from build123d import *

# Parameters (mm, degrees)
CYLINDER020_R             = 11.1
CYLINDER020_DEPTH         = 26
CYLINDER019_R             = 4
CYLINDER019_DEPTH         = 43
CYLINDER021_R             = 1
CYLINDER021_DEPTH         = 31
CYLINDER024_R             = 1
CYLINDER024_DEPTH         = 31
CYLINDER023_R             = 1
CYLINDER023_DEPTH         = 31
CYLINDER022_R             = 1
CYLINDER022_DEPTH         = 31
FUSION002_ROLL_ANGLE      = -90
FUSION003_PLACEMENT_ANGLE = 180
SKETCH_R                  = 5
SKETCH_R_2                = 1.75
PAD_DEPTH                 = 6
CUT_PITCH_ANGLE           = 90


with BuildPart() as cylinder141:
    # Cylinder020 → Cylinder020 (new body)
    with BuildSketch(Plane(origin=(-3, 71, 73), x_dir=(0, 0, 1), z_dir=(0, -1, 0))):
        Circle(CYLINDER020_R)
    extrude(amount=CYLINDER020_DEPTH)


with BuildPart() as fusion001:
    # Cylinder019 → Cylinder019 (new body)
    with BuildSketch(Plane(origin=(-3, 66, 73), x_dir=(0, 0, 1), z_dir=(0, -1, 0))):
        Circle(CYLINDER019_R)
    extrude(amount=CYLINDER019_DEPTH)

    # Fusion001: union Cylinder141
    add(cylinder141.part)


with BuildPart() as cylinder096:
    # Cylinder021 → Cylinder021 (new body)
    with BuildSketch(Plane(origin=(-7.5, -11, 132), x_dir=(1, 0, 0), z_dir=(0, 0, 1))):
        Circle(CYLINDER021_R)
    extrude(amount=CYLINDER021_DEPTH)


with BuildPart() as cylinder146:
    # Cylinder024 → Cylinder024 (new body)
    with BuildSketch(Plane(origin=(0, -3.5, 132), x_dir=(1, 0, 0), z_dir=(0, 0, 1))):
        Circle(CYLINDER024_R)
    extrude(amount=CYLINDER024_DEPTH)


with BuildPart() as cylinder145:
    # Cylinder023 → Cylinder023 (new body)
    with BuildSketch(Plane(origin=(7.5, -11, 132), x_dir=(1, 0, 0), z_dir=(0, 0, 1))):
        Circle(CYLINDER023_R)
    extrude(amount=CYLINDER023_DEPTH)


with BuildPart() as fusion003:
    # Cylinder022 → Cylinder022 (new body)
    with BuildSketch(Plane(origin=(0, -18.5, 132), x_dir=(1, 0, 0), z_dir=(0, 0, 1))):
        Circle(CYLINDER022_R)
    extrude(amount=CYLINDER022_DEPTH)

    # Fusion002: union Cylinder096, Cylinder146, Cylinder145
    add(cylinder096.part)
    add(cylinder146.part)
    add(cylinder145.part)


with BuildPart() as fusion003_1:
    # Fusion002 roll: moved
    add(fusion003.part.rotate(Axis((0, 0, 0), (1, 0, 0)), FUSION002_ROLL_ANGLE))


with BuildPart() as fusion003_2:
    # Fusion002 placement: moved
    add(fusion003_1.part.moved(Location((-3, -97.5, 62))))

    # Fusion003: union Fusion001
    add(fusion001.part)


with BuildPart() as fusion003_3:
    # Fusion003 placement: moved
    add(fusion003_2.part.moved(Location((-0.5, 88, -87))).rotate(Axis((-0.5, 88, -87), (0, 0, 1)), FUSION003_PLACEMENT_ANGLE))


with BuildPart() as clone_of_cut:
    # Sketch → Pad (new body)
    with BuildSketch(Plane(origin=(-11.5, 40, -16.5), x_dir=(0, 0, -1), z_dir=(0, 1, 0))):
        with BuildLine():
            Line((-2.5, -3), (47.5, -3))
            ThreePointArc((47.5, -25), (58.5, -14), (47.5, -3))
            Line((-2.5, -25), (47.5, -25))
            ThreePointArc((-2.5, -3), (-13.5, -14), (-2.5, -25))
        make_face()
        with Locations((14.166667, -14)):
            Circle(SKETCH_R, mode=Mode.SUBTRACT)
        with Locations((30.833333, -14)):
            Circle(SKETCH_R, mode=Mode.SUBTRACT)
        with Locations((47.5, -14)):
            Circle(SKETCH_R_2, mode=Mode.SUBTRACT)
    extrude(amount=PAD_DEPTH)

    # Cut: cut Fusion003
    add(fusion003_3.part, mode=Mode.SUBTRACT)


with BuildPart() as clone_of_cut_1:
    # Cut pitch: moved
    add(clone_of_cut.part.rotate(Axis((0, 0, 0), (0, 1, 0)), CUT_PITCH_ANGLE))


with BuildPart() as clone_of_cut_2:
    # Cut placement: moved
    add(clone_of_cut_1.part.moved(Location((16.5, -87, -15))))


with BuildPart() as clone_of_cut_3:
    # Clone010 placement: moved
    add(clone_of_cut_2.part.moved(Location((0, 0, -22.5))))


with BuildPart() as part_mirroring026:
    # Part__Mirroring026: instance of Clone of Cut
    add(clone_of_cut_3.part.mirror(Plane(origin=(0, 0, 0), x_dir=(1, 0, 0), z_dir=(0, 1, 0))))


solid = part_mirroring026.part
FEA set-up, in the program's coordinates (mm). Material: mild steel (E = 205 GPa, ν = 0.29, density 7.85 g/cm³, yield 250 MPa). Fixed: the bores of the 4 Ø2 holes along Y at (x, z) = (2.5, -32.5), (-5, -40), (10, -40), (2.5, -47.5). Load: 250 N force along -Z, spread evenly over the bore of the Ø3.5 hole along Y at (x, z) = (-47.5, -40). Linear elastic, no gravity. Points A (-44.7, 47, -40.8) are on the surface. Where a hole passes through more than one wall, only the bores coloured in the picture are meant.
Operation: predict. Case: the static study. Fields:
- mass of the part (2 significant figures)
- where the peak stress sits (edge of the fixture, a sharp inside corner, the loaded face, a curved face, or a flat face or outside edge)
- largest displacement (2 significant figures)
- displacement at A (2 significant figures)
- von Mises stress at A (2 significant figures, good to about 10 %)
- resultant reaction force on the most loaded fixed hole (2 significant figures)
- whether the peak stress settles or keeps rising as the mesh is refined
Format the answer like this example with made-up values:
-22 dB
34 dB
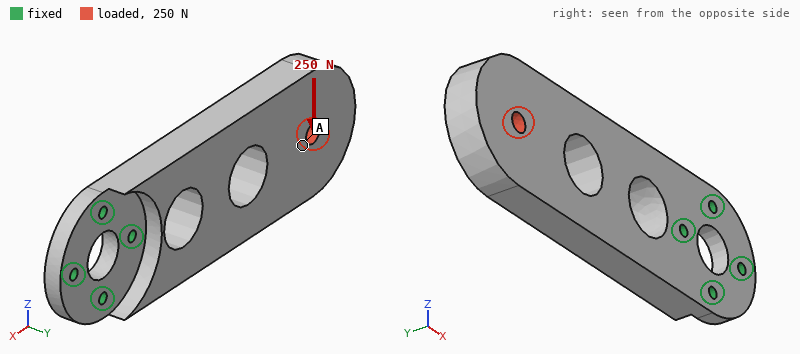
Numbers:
51 g
edge of the fixture
22 µm
15 µm
7.5 MPa
550 N
keeps rising
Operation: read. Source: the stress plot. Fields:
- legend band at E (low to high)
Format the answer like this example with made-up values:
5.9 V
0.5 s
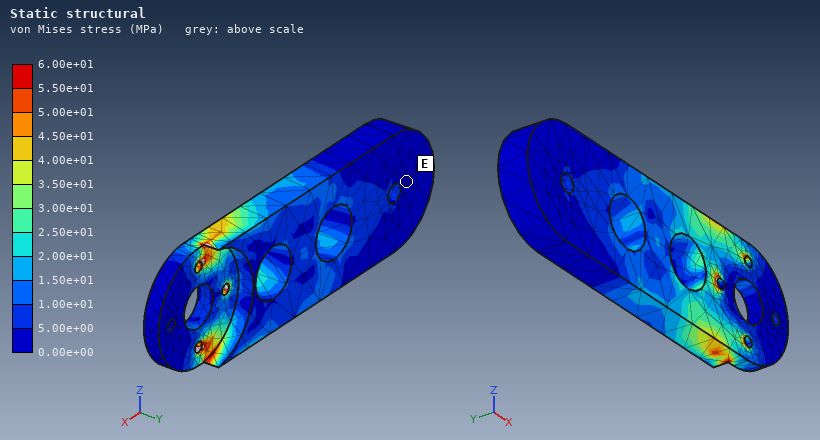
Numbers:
0.00e+00 to 5.00e+00 MPa
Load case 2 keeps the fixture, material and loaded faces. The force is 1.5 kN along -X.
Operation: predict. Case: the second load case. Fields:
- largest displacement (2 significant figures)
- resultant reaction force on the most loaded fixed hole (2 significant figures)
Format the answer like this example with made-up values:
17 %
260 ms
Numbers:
35 µm
520 N
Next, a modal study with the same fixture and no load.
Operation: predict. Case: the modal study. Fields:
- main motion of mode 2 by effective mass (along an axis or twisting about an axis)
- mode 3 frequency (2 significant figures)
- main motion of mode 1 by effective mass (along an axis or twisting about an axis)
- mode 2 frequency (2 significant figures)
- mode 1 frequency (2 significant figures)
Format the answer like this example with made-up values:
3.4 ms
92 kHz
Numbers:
along Z
4900 Hz
along Y
3900 Hz
1100 Hz
